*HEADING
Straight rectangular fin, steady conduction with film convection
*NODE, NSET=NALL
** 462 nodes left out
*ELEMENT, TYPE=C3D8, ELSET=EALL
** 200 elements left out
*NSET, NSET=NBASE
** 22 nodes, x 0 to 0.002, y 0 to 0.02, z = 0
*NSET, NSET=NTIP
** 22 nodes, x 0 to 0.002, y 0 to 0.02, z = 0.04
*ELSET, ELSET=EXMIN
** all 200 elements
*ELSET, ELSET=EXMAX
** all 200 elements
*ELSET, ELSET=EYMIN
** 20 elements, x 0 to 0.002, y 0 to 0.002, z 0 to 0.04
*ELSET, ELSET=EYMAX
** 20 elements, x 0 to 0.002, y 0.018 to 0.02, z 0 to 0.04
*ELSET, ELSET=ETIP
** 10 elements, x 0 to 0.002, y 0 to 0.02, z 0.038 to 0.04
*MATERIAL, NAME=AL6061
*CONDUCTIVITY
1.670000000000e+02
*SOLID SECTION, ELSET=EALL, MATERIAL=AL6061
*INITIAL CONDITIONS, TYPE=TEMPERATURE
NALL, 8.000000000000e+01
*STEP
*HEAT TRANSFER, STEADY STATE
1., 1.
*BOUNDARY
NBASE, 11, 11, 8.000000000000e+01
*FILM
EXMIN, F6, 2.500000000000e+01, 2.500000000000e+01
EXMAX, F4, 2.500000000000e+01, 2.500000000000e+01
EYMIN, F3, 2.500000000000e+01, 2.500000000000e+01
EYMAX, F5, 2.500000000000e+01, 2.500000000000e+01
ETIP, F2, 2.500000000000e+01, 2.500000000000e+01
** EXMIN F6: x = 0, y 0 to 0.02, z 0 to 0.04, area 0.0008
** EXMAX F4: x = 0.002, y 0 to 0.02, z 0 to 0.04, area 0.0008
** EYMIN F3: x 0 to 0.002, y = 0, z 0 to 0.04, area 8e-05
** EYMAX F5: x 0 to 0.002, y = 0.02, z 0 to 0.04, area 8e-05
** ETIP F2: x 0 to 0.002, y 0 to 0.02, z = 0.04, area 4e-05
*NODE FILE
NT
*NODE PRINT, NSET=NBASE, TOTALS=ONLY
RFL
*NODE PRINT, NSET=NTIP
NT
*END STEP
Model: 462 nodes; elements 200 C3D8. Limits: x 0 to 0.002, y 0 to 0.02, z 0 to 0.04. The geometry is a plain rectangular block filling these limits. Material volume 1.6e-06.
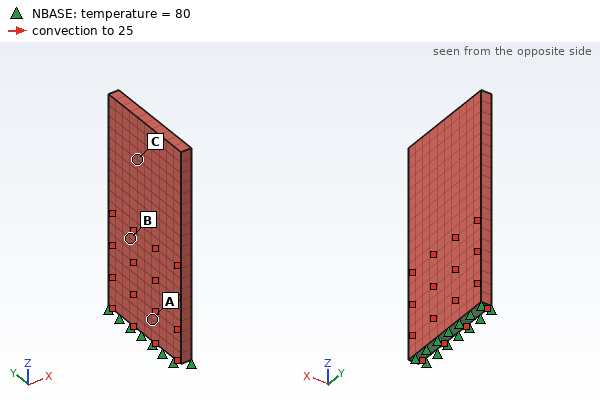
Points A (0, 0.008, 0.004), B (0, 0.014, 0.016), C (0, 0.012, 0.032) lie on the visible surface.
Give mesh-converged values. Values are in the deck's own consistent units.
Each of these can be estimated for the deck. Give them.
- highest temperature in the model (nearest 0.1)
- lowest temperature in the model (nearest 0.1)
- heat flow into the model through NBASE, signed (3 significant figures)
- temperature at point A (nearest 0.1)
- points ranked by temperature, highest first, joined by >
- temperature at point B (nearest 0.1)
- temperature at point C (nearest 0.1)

80.0
73.2
2.25
78.7
A > B > C
75.7
73.5
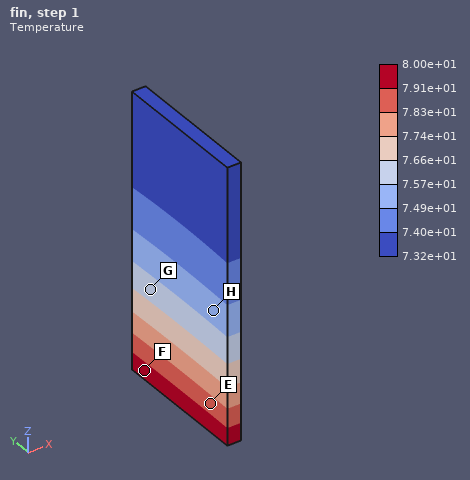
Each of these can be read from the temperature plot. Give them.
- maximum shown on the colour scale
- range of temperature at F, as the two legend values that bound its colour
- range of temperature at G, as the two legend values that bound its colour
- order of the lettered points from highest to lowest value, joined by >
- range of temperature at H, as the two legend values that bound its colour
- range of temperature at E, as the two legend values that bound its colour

8.00e+01
7.91e+01 to 8.00e+01
7.57e+01 to 7.66e+01
F > E > G > H
7.49e+01 to 7.57e+01
7.83e+01 to 7.91e+01
